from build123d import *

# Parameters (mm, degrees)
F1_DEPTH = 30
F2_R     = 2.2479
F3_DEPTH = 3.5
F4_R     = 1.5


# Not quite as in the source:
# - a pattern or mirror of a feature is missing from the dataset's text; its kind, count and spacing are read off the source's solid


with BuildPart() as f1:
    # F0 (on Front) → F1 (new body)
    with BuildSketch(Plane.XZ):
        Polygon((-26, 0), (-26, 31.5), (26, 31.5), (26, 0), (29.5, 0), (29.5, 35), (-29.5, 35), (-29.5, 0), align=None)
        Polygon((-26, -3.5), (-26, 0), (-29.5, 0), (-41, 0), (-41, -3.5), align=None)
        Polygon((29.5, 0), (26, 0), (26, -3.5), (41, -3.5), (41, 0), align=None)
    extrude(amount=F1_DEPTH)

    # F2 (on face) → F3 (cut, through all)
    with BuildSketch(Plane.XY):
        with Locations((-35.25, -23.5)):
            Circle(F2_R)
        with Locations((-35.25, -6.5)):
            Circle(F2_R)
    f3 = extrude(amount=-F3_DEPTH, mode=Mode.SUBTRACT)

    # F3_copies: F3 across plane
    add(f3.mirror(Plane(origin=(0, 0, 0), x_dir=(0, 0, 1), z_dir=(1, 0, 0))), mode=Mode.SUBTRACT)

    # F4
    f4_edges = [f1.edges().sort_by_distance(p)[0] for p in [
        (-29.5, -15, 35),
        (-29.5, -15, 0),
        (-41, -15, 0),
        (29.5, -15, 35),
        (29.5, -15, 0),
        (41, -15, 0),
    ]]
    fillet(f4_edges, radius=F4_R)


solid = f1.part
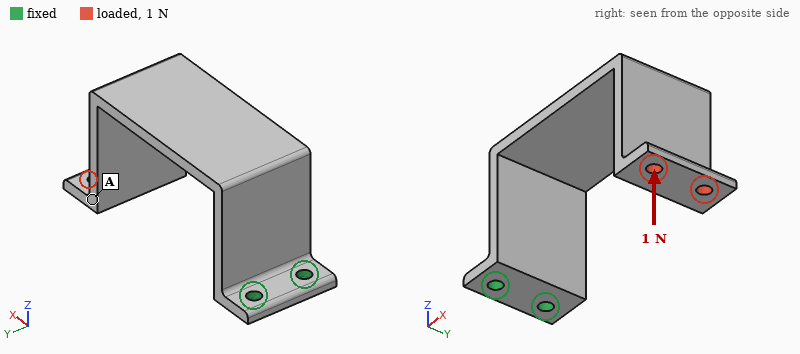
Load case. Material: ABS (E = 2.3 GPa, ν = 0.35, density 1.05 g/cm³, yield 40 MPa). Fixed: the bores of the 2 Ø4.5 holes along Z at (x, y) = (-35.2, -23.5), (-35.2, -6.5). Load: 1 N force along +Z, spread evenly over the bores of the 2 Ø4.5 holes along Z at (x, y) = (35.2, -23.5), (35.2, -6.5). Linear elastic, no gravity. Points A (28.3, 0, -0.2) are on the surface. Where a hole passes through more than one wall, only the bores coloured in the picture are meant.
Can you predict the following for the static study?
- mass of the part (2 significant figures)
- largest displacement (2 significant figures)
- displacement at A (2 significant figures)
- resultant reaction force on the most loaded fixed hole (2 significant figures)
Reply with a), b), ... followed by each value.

a) 16 g
b) 1.1 mm
c) 0.88 mm
d) 0.88 N
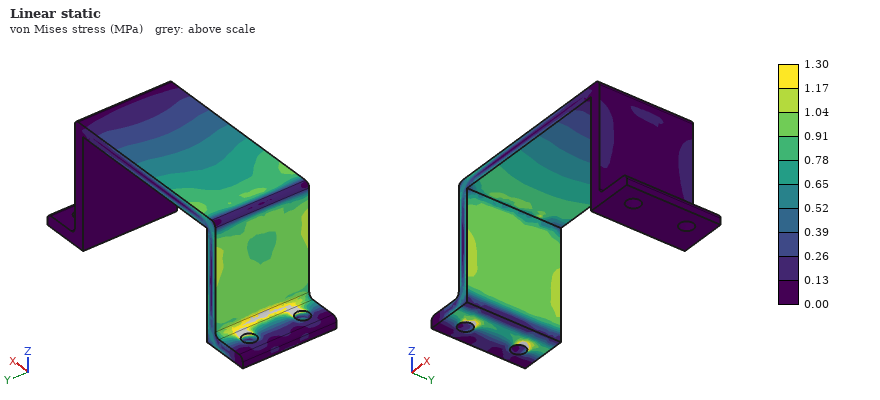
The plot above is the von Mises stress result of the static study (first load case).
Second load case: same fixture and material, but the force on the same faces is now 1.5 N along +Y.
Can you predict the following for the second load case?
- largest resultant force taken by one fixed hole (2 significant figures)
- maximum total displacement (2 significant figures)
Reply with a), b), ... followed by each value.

a) 5.3 N
b) 0.87 mm
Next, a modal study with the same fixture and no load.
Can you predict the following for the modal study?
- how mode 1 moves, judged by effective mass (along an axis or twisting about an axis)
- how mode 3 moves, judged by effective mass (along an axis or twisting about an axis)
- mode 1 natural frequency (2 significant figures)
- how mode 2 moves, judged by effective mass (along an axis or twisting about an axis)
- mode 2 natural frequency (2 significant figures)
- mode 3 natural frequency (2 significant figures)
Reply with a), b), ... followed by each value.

a) along Z
b) along X
c) 67 Hz
d) along Y
e) 110 Hz
f) 180 Hz
